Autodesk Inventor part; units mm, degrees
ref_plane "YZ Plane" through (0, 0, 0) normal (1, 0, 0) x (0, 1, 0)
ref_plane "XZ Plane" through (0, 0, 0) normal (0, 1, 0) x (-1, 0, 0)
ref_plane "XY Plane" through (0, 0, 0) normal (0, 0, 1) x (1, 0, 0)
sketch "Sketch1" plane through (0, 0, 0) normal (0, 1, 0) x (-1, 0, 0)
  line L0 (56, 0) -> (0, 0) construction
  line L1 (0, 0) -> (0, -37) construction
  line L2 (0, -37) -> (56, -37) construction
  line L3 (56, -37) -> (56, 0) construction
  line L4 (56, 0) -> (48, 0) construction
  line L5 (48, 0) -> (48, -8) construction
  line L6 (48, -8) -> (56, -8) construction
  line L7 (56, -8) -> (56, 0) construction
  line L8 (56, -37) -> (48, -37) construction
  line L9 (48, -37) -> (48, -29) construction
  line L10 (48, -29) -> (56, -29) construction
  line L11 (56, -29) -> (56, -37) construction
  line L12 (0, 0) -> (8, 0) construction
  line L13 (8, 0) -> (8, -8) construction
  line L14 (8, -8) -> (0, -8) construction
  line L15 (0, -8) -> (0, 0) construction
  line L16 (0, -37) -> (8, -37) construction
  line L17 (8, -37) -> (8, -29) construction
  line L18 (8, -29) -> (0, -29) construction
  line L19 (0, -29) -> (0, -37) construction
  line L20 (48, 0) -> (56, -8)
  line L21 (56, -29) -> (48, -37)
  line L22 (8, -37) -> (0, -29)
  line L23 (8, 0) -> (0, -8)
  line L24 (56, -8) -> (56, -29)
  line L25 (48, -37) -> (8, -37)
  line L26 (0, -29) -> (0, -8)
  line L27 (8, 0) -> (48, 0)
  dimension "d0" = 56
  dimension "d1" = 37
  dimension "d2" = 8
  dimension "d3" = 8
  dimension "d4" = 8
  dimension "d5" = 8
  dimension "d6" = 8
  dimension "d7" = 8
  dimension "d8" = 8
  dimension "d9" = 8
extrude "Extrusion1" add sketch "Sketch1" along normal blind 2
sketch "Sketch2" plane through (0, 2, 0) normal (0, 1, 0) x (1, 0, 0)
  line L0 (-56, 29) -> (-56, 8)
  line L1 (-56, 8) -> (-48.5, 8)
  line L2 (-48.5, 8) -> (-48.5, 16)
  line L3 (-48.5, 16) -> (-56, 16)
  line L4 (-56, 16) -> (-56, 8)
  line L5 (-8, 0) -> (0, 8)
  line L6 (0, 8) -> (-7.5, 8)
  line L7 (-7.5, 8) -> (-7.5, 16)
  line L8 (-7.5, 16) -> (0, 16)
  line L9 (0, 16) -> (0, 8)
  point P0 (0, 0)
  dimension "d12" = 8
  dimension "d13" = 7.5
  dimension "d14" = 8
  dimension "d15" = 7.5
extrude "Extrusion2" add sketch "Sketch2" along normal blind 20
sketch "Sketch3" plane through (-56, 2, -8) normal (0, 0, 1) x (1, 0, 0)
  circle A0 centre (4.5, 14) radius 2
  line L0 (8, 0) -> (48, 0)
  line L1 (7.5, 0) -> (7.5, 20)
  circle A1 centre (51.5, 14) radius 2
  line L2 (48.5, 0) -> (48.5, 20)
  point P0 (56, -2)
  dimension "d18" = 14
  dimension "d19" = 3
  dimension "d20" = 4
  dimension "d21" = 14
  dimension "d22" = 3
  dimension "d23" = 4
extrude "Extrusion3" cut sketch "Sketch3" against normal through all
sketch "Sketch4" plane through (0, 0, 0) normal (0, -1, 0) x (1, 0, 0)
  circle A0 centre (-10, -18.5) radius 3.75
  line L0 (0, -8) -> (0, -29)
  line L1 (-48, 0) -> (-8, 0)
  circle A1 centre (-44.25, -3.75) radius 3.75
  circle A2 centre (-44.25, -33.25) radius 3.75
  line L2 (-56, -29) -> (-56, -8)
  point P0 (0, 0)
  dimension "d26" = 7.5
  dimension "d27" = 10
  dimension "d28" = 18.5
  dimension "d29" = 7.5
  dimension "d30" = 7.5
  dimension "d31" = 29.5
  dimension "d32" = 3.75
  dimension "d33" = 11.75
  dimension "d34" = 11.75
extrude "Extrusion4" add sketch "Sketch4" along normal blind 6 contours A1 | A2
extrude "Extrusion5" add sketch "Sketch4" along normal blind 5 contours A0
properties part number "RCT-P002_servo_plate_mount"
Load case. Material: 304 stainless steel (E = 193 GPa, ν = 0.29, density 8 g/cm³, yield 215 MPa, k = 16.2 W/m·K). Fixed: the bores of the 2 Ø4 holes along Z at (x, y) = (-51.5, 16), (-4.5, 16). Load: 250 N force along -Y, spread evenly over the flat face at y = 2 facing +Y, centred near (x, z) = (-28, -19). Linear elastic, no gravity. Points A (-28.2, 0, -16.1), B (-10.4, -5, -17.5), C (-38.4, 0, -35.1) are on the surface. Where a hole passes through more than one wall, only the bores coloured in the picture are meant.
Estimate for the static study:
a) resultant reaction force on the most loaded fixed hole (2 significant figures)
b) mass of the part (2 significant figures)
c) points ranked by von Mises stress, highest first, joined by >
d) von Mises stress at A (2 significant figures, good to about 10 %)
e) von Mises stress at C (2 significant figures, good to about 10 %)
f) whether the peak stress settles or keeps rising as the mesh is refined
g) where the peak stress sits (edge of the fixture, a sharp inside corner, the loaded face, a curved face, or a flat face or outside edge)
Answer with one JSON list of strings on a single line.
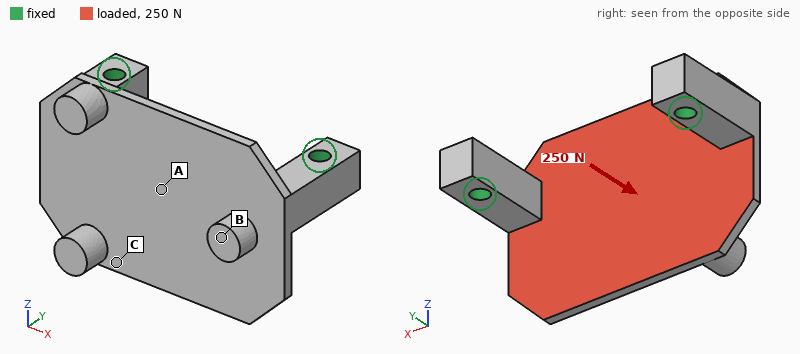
["150 N", "55 g", "A > C > B", "28 MPa", "14 MPa", "keeps rising", "a sharp inside corner"]
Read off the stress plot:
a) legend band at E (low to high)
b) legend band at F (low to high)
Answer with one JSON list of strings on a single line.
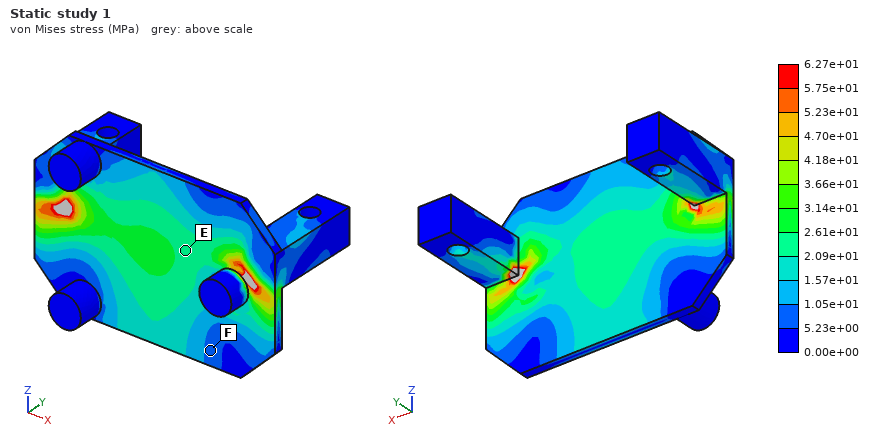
["2.09e+01 to 2.61e+01 MPa", "5.23e+00 to 1.05e+01 MPa"]
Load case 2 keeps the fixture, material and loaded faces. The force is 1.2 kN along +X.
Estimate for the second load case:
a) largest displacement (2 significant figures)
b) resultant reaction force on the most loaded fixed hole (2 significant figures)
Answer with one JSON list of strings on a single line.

["22 µm", "620 N"]
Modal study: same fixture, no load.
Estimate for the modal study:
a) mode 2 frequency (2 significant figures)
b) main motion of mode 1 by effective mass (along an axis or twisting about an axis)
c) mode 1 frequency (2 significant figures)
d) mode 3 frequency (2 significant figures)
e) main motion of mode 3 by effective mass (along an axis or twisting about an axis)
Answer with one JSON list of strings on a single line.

["4200 Hz", "along Y", "2100 Hz", "4600 Hz", "along Y"]
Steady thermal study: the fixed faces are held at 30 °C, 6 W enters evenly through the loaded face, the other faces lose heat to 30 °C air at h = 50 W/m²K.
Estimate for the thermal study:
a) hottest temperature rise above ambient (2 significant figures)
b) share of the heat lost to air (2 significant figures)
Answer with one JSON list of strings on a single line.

["35 K", "65 %"]
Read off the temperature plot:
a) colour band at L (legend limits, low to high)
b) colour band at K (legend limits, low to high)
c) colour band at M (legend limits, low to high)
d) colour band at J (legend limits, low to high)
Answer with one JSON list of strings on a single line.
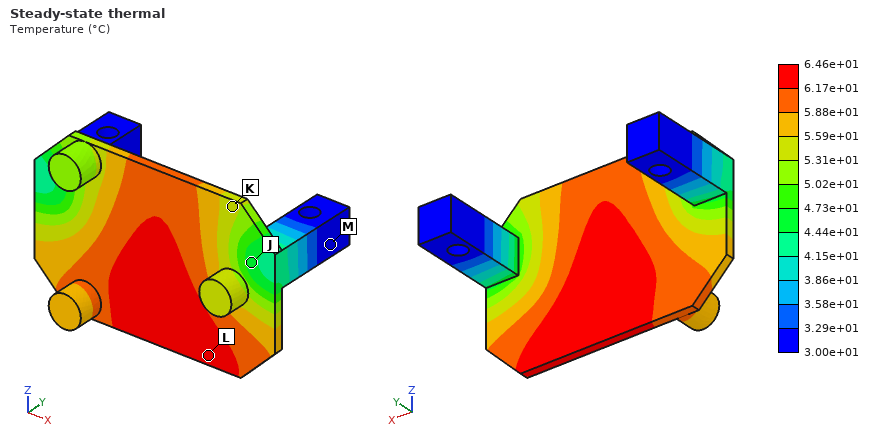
["6.17e+01 to 6.46e+01 °C", "5.31e+01 to 5.59e+01 °C", "3.00e+01 to 3.29e+01 °C", "4.44e+01 to 4.73e+01 °C"]
